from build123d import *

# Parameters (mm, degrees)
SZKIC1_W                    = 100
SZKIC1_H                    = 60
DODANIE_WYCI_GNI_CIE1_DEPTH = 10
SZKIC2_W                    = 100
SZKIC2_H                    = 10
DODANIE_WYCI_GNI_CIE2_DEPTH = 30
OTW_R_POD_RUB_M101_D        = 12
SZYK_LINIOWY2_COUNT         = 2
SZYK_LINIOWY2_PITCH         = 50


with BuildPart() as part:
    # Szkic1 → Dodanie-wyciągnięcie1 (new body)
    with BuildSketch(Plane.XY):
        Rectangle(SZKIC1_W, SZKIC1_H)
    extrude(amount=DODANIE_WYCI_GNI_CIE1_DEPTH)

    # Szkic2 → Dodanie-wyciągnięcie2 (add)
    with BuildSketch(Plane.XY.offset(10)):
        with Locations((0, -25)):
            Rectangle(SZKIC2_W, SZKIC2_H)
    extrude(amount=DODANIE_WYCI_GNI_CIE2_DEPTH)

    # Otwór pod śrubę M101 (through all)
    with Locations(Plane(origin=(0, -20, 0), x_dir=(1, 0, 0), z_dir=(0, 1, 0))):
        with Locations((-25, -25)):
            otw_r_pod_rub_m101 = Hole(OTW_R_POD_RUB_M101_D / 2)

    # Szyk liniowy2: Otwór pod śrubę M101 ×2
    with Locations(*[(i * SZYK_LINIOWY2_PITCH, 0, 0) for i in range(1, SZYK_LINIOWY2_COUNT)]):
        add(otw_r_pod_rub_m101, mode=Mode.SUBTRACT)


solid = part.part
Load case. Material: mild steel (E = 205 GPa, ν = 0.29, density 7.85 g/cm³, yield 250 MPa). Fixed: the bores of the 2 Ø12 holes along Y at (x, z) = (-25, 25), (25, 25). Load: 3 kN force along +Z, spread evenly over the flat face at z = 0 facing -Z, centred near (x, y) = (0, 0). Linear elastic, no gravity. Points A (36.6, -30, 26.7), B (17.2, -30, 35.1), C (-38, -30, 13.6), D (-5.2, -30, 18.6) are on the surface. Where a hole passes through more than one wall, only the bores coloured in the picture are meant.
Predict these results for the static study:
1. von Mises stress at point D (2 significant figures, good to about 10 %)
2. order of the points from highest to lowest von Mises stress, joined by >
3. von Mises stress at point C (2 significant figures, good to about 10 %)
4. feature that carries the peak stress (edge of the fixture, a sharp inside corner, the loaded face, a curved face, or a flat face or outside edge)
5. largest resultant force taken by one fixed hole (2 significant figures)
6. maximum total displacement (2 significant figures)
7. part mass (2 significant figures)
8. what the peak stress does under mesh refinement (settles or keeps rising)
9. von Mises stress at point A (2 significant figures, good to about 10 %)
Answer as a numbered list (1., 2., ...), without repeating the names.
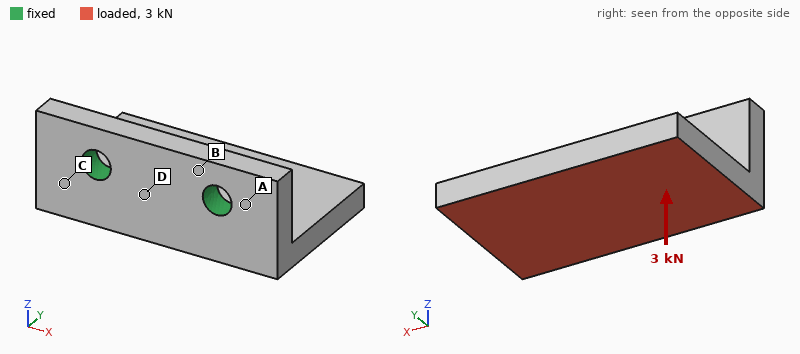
1. 27 MPa
2. C > D > A > B
3. 33 MPa
4. edge of the fixture
5. 1.5 kN
6. 71 µm
7. 690 g
8. keeps rising
9. 14 MPa
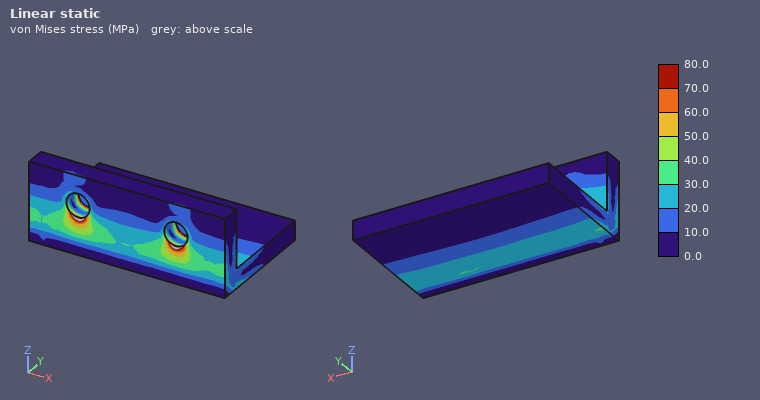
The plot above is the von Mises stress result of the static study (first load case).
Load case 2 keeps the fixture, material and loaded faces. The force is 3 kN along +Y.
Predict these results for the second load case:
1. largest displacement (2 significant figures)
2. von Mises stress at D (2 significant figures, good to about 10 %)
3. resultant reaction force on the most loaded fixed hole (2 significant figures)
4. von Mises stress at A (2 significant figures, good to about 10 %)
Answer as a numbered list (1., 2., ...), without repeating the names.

1. 35 µm
2. 16 MPa
3. 1.5 kN
4. 13 MPa
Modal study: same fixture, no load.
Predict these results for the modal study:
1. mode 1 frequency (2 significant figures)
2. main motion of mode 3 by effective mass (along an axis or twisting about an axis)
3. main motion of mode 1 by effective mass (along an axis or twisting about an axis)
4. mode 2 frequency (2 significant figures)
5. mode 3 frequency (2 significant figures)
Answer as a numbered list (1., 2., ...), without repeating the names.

1. 1800 Hz
2. along X
3. along Z
4. 3300 Hz
5. 5100 Hz
